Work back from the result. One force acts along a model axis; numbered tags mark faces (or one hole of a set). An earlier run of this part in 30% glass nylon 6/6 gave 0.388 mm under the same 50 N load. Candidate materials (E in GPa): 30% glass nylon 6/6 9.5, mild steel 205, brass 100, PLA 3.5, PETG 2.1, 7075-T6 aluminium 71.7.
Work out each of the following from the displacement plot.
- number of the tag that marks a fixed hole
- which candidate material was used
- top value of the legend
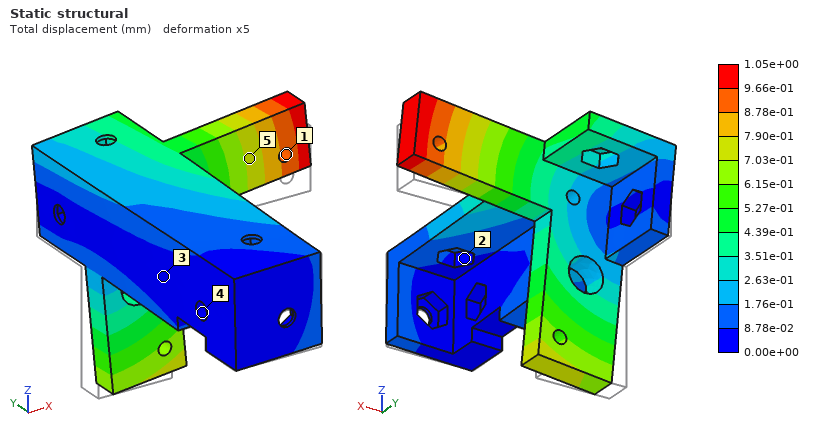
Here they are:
4
PLA
1.05e+00 mm
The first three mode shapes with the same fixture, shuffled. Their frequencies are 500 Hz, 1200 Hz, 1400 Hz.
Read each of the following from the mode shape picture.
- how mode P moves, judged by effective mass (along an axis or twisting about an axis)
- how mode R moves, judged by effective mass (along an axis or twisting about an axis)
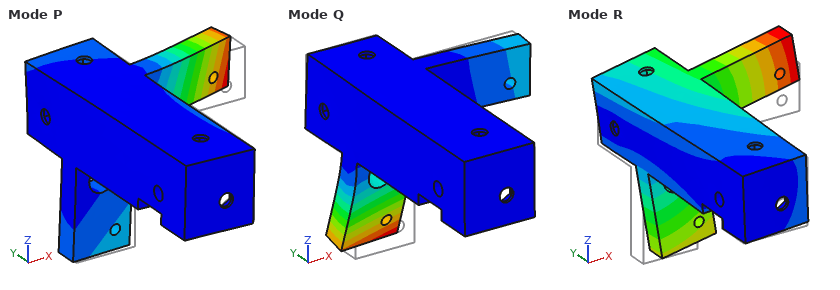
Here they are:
along Y
along Z
